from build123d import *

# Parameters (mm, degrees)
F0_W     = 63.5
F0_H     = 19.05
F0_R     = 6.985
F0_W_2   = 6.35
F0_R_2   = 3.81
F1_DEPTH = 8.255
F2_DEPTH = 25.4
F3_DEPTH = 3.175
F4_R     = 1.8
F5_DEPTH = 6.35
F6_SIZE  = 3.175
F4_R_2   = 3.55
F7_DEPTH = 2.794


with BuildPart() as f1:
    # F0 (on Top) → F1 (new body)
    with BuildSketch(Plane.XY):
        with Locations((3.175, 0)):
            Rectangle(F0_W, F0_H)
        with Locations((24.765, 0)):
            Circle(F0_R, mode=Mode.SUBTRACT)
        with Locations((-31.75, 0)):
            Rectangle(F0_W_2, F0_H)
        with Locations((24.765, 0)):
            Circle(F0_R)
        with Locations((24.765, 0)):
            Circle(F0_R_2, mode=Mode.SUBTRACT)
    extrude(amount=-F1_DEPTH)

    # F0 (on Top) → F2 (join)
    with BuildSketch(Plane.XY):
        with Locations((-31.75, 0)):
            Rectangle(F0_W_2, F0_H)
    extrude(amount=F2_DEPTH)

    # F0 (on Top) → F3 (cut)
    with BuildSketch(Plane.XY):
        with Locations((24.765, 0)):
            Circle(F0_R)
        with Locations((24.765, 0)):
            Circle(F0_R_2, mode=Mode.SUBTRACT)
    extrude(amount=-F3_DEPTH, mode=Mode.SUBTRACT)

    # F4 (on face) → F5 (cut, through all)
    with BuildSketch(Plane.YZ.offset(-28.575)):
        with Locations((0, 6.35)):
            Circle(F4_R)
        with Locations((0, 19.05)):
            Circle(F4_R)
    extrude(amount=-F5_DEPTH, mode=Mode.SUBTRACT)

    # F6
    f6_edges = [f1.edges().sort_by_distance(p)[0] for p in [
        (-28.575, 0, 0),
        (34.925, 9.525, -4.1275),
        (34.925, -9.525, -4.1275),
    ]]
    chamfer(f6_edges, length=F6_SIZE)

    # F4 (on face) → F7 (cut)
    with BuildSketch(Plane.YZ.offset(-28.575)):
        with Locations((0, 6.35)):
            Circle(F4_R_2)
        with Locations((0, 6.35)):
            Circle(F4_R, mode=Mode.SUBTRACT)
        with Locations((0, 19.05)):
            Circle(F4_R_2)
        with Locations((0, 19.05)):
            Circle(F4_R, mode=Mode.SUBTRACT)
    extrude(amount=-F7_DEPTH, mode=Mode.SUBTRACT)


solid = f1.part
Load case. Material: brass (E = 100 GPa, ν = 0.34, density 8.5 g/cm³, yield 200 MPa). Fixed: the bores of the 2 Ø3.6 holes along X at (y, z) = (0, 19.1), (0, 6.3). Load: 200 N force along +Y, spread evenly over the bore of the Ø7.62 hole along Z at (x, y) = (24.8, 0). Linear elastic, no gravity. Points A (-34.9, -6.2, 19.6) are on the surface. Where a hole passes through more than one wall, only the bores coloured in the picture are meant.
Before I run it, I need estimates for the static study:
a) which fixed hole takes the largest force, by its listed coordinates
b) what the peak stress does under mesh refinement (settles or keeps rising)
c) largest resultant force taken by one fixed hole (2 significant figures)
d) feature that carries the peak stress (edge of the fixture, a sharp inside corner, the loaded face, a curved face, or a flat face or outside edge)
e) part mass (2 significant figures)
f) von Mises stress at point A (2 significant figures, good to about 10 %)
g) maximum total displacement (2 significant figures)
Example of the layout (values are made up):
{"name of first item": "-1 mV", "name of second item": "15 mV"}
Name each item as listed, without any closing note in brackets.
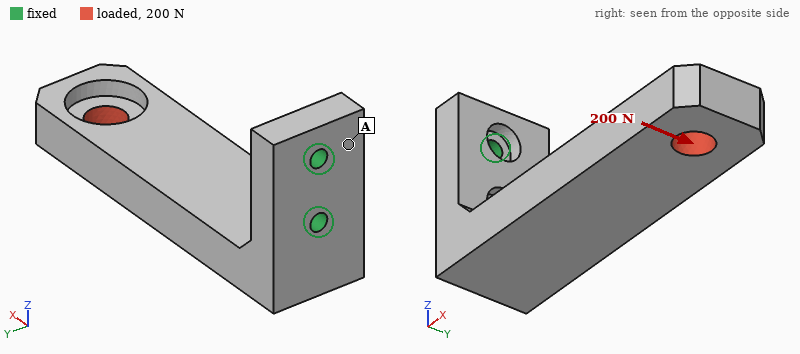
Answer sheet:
{"which fixed hole takes the largest force, by its listed coordinates": "(0, 6.3)", "what the peak stress does under mesh refinement": "keeps rising", "largest resultant force taken by one fixed hole": "280 N", "feature that carries the peak stress": "edge of the fixture", "part mass": "110 g", "von Mises stress at point A": "21 MPa", "maximum total displacement": "0.23 mm"}
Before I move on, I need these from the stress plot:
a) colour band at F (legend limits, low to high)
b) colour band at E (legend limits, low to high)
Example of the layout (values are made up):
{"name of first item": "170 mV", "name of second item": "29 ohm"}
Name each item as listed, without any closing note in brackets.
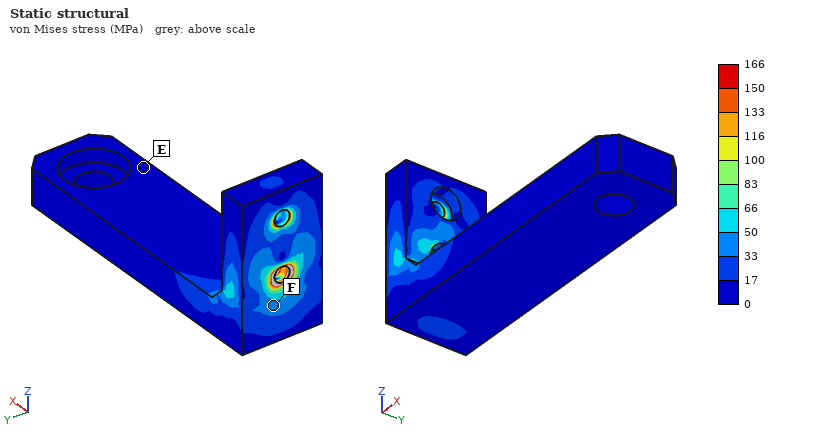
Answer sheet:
{"colour band at F": "33 to 50 MPa", "colour band at E": "0 to 17 MPa"}
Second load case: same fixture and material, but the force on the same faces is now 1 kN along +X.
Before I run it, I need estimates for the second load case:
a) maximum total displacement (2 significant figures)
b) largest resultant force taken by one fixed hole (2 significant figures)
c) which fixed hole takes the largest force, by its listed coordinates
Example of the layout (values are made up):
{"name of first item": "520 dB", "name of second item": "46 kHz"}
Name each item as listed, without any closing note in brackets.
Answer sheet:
{"maximum total displacement": "0.22 mm", "largest resultant force taken by one fixed hole": "1.6 kN", "which fixed hole takes the largest force, by its listed coordinates": "(0, 6.3)"}
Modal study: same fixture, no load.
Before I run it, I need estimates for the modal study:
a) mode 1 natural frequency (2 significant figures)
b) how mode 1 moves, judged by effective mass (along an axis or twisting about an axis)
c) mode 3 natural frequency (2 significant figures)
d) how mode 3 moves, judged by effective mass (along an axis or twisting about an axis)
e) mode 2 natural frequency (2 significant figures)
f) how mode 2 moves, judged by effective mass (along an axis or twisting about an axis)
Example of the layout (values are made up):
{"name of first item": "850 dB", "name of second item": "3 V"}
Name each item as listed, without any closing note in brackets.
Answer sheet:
{"mode 1 natural frequency": "730 Hz", "how mode 1 moves, judged by effective mass": "along Z", "mode 3 natural frequency": "4100 Hz", "how mode 3 moves, judged by effective mass": "along X", "mode 2 natural frequency": "870 Hz", "how mode 2 moves, judged by effective mass": "along Y"}
